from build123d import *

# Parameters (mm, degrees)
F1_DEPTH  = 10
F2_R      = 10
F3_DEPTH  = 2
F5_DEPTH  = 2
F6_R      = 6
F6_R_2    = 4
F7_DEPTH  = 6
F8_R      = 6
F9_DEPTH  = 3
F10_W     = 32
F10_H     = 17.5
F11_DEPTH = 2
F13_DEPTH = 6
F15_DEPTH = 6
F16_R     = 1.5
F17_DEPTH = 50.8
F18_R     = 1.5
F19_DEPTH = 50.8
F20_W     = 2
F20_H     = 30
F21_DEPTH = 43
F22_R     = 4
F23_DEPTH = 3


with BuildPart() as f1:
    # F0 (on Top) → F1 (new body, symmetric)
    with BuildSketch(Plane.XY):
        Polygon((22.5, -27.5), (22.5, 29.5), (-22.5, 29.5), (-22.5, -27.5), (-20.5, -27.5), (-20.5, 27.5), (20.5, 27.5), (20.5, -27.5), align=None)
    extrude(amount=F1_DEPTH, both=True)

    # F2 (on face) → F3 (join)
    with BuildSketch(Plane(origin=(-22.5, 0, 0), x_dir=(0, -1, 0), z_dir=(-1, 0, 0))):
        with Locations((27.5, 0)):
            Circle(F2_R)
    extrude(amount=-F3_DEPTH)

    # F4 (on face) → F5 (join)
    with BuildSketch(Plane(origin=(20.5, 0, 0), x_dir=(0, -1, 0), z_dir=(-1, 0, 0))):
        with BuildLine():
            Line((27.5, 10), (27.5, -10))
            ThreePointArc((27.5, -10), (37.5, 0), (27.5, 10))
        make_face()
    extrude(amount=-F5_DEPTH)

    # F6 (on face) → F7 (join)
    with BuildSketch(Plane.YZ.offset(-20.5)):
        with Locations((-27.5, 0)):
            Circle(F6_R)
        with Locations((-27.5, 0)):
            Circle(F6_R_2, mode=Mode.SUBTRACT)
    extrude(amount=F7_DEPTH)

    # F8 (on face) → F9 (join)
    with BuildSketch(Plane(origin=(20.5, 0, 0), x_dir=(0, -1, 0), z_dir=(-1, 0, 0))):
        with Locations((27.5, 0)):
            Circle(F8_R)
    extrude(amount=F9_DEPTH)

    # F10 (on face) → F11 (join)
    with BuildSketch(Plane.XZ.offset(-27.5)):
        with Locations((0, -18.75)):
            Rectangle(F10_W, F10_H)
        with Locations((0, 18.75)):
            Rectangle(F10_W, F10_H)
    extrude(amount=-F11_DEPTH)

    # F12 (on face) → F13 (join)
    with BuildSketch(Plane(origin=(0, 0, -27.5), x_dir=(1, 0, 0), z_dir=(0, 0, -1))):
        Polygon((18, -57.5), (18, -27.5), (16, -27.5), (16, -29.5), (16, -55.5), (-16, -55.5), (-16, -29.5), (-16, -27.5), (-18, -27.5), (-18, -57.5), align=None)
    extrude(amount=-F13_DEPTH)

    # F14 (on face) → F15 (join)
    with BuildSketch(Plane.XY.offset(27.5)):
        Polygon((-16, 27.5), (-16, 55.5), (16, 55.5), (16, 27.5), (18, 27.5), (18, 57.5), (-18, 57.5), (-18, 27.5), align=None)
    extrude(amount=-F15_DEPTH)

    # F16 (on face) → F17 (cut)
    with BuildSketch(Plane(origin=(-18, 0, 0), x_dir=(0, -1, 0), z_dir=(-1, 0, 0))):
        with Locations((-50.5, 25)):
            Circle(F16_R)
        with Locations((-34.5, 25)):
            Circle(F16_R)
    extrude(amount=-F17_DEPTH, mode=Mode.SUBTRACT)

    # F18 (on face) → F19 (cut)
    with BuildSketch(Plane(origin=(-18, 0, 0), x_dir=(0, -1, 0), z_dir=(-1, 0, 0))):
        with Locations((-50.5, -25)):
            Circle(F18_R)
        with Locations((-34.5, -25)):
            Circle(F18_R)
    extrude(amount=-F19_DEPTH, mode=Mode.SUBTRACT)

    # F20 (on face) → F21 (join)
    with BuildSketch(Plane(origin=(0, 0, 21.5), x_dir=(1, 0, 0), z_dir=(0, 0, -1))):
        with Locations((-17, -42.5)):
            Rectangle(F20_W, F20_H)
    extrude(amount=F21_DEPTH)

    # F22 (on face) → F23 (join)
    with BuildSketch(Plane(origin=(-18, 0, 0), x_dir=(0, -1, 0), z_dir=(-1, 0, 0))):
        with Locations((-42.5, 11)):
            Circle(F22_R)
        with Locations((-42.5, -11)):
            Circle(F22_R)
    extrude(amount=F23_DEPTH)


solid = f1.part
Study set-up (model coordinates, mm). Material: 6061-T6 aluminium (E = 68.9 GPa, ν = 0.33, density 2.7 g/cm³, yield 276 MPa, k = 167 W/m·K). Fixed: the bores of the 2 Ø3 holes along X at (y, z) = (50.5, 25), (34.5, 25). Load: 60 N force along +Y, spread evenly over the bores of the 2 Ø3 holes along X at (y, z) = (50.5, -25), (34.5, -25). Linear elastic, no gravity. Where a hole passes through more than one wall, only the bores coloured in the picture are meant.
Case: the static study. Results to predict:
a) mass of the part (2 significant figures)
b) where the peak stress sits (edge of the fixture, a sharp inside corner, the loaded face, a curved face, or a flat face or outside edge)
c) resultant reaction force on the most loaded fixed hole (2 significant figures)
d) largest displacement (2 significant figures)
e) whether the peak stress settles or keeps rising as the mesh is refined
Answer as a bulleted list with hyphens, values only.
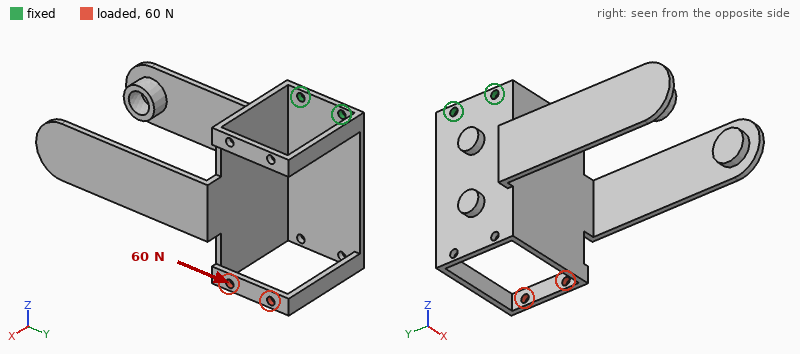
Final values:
- 40 g
- edge of the fixture
- 190 N
- 1.2 mm
- keeps rising
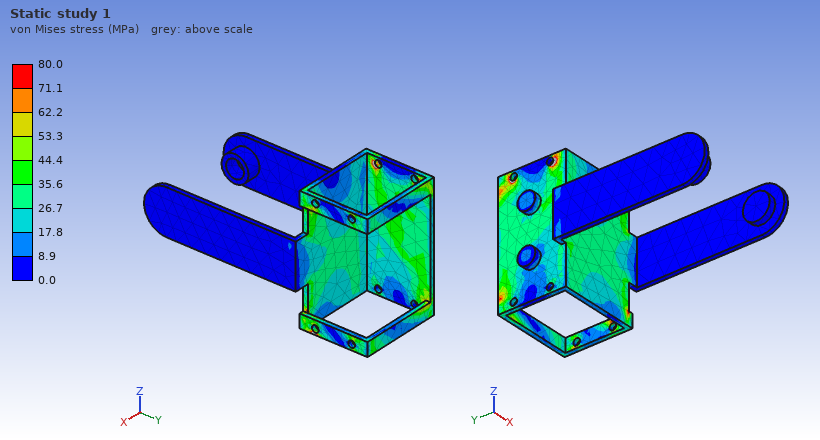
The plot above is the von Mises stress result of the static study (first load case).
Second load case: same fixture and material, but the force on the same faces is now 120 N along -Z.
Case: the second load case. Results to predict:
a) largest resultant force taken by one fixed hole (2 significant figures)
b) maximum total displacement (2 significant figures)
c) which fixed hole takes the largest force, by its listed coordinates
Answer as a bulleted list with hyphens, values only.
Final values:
- 82 N
- 1.4 mm
- (50.5, 25)
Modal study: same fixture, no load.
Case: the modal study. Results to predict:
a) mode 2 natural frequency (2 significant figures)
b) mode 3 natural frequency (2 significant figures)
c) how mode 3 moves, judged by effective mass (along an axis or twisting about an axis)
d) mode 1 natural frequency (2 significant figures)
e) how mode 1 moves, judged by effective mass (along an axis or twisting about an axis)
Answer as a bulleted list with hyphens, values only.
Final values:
- 280 Hz
- 360 Hz
- along Z
- 210 Hz
- along X
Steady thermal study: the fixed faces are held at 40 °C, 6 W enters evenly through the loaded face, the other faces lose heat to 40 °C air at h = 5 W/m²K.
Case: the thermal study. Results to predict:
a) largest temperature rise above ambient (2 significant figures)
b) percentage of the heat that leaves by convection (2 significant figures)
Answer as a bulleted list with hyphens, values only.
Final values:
- 54 K
- 15 %
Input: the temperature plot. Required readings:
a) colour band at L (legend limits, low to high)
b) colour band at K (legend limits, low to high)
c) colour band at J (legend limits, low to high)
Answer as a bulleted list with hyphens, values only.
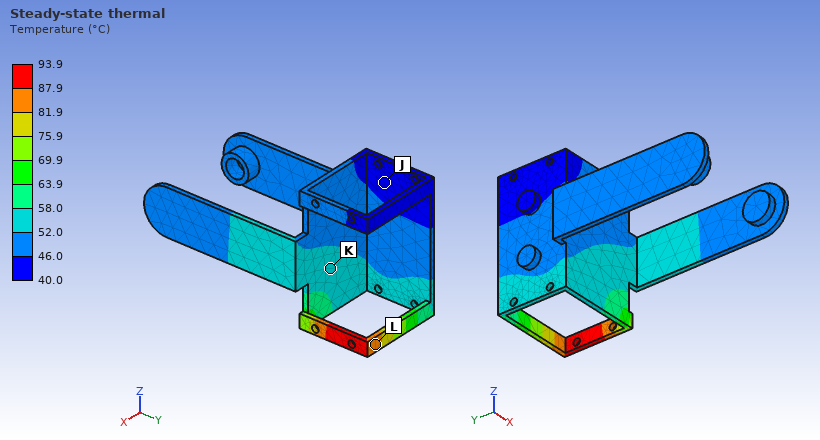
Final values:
- 81.9 to 87.9 °C
- 52.0 to 58.0 °C
- 40.0 to 46.0 °C
